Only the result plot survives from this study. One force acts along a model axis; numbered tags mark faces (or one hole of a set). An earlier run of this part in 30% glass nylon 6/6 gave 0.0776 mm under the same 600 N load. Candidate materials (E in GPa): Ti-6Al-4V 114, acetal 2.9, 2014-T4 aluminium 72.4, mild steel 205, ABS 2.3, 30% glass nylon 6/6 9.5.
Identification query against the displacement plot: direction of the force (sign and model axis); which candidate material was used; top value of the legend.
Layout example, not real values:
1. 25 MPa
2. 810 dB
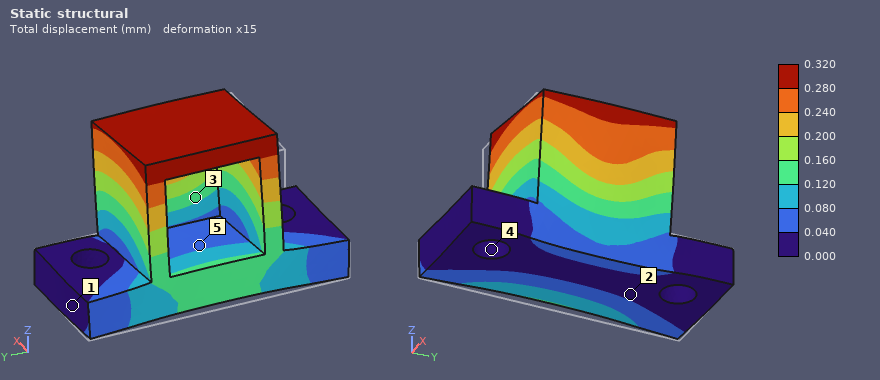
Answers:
1. +X
2. ABS
3. 0.320 mm
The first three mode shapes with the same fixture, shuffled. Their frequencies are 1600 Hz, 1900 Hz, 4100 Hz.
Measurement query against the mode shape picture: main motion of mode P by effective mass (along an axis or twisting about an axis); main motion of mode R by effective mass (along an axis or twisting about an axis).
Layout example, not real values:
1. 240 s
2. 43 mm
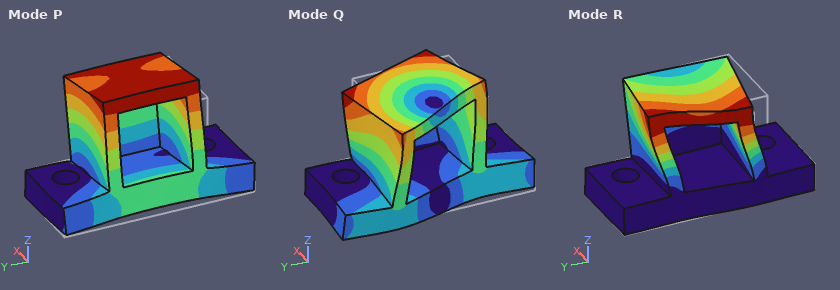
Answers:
1. along X
2. along Y
